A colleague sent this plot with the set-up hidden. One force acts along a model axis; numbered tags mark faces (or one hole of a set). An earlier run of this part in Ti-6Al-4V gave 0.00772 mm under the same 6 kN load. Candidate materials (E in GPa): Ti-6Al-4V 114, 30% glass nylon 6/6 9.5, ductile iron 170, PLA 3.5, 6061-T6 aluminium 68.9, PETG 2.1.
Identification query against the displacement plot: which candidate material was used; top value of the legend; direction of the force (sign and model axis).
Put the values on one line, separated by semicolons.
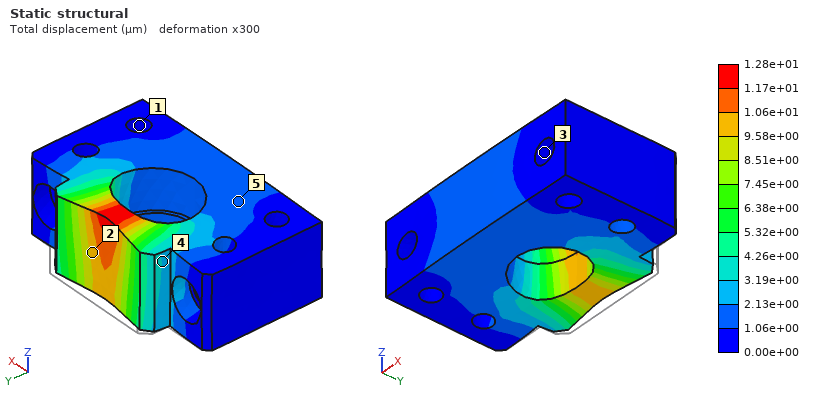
6061-T6 aluminium; 1.28e+01 µm; -Y
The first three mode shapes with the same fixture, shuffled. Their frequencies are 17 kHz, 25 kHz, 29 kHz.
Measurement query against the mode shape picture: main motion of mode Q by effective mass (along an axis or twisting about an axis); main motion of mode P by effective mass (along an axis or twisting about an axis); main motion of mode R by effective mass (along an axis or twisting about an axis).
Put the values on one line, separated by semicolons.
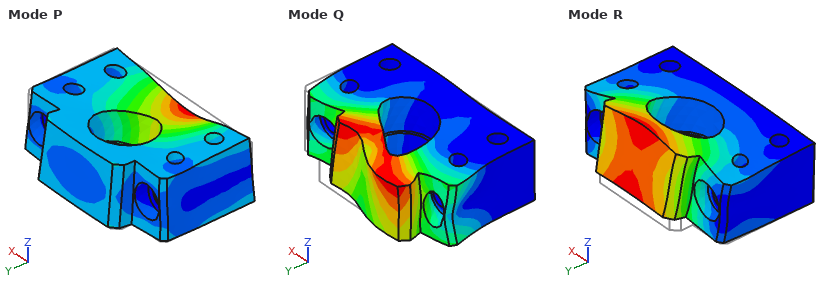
along X; along Z; along Z
